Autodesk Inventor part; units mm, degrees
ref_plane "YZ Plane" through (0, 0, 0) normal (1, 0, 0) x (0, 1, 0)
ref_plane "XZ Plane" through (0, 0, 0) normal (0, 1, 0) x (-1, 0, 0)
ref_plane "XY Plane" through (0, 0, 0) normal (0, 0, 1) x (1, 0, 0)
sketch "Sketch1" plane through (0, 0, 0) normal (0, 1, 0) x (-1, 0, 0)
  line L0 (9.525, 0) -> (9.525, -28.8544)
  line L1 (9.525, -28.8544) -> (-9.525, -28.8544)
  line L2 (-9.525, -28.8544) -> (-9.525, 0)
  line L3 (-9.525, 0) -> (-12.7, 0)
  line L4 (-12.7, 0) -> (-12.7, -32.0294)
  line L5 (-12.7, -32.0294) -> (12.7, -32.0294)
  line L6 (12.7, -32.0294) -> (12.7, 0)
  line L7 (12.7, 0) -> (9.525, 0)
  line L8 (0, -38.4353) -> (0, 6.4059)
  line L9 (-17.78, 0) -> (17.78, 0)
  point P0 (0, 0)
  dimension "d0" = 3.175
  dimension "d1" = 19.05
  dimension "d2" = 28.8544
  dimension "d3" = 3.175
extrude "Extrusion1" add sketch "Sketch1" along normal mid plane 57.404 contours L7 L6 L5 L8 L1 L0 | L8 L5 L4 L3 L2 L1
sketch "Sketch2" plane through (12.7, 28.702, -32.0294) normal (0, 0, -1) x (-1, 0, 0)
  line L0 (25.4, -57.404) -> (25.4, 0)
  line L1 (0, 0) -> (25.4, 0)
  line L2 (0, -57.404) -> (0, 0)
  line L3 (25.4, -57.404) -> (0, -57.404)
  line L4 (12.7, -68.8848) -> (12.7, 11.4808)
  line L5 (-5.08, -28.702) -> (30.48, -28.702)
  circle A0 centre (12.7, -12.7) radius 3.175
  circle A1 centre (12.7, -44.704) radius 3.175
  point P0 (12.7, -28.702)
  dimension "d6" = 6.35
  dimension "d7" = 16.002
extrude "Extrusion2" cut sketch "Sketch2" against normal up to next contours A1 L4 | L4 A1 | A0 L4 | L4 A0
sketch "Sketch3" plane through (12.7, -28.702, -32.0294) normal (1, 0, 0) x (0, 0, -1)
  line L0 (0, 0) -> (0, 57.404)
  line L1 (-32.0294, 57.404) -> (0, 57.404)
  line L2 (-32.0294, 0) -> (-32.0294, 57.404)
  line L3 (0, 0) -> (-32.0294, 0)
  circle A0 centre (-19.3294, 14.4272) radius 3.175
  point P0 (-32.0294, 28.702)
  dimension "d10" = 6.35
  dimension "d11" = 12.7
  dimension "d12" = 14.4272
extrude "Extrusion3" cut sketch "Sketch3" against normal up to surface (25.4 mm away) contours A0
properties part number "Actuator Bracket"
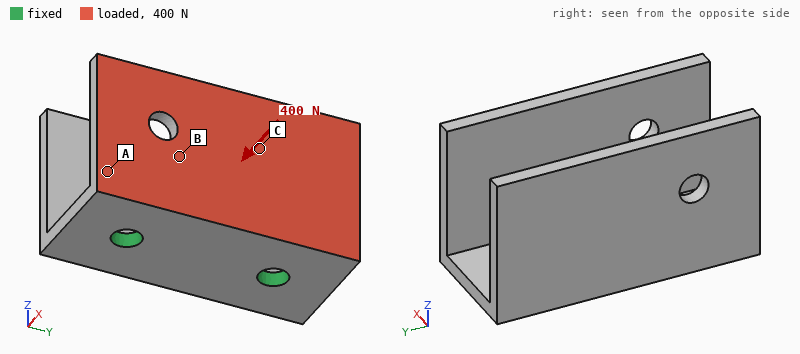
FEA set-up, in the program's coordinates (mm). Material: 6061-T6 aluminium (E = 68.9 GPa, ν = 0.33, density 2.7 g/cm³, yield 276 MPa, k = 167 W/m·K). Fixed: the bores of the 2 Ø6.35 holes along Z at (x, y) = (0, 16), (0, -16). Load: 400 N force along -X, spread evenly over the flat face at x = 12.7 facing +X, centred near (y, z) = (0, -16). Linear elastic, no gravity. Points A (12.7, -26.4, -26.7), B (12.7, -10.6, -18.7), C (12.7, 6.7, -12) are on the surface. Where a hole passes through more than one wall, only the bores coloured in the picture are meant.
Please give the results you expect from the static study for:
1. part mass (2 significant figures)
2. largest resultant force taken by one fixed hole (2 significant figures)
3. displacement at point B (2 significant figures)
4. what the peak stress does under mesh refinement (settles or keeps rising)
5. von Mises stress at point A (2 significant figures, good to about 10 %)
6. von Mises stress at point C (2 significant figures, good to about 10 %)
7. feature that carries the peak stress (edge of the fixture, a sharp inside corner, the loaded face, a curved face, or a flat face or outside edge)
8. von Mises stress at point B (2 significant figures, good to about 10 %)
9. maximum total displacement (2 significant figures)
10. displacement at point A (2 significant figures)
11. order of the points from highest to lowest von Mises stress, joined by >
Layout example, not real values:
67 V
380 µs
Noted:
40 g
200 N
0.089 mm
keeps rising
41 MPa
8.7 MPa
edge of the fixture
21 MPa
0.26 mm
0.041 mm
A > B > C
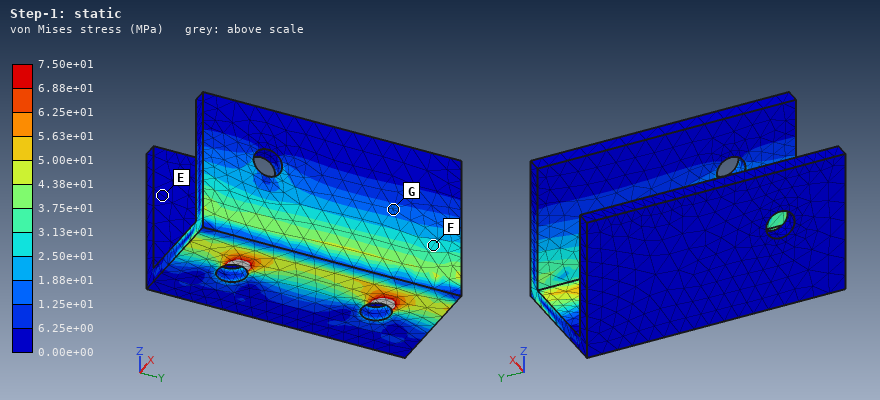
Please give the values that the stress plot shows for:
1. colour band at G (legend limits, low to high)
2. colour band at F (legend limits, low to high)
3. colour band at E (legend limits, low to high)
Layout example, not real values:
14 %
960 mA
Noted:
1.25e+01 to 1.88e+01 MPa
2.50e+01 to 3.13e+01 MPa
0.00e+00 to 6.25e+00 MPa
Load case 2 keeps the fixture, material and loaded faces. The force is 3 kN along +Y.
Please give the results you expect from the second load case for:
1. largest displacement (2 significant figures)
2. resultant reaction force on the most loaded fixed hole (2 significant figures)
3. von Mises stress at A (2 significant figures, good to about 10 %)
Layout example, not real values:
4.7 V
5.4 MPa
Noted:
0.17 mm
2.1 kN
46 MPa
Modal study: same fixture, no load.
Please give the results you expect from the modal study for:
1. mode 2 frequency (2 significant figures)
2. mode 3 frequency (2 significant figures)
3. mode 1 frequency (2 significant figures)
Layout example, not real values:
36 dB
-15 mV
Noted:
2000 Hz
3400 Hz
1900 Hz
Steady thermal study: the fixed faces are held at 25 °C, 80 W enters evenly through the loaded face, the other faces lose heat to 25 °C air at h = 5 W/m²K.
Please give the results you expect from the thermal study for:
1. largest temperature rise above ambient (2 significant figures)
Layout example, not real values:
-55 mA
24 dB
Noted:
68 K
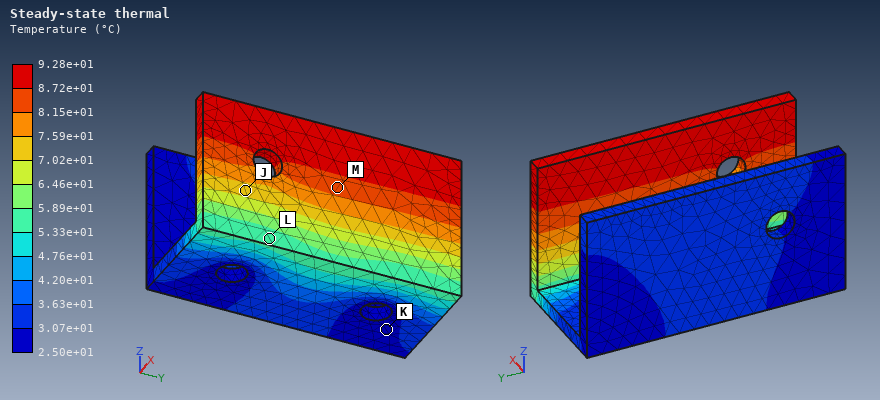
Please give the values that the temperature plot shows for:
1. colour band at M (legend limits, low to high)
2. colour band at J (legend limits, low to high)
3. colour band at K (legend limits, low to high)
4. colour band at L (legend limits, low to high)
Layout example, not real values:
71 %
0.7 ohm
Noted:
8.15e+01 to 8.72e+01 °C
7.02e+01 to 7.59e+01 °C
2.50e+01 to 3.07e+01 °C
5.33e+01 to 5.89e+01 °C
